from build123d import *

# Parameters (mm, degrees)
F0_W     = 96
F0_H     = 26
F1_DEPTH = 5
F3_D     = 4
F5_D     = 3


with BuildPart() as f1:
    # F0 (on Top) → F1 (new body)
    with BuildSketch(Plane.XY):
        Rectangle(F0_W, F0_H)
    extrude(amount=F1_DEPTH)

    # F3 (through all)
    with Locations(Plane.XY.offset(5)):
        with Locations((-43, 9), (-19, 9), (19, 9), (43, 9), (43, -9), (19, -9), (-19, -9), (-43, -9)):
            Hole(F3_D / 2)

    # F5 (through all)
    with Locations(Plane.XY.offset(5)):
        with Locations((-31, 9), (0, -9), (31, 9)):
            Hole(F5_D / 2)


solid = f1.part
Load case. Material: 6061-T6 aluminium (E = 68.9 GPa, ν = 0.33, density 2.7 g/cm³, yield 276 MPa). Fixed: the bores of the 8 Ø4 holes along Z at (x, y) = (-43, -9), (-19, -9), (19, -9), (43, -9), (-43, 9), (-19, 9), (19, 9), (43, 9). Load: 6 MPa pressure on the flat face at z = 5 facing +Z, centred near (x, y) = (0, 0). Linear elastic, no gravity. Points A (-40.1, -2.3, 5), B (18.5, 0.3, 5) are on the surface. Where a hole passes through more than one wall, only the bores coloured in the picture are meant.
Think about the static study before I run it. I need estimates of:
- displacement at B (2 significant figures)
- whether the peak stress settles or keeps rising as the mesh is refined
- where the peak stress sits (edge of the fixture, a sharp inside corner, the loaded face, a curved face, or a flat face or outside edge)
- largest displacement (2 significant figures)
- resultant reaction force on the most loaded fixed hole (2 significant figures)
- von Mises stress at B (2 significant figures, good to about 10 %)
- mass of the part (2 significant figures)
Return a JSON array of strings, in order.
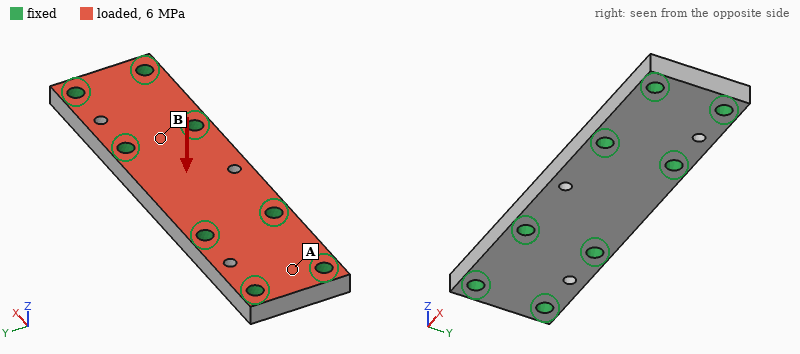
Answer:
["8.0 µm", "keeps rising", "edge of the fixture", "52 µm", "2.4 kN", "63 MPa", "32 g"]
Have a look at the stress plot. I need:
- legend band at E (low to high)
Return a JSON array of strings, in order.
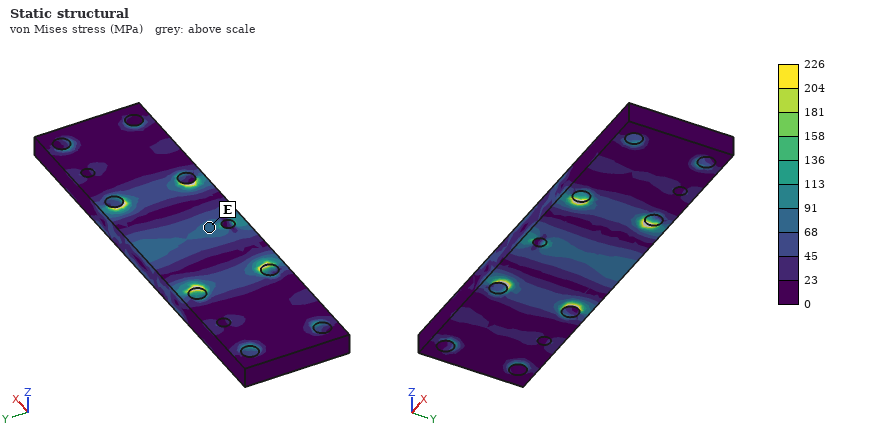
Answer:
["68 to 91 MPa"]
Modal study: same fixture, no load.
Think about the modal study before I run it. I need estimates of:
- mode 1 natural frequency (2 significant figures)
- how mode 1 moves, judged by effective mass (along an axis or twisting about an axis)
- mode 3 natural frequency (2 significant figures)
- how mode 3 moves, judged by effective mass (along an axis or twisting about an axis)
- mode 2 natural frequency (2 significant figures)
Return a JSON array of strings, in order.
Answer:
["17 kHz", "along Z", "36 kHz", "along Y", "23 kHz"]
